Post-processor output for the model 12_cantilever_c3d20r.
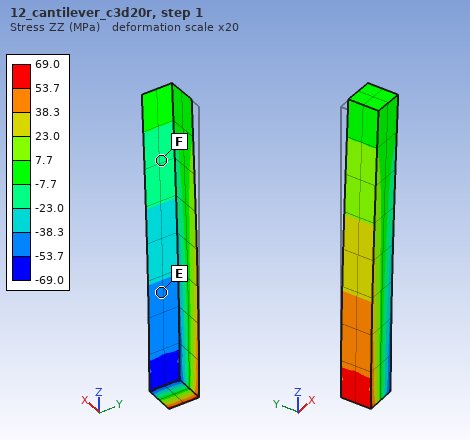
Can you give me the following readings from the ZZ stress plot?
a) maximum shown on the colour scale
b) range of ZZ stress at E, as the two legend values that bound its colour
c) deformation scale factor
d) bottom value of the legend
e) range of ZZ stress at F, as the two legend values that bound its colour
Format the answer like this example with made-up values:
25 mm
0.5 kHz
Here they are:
69.0 MPa
-53.7 to -38.3 MPa
20
-69.0 MPa
-23.0 to -7.7 MPa
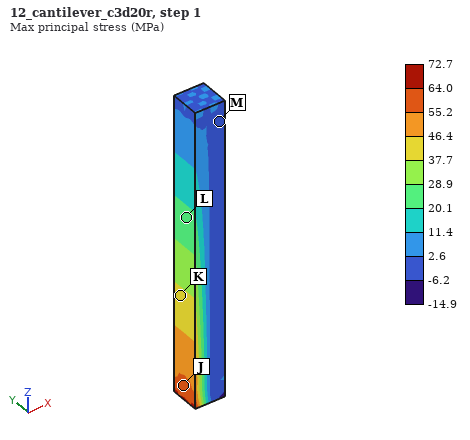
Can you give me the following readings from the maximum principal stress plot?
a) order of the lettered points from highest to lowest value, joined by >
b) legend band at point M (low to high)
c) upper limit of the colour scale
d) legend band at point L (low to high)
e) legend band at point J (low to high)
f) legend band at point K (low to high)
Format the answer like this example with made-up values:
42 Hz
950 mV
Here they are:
J > K > L > M
-6.2 to 2.6 MPa
72.7 MPa
20.1 to 28.9 MPa
55.2 to 64.0 MPa
37.7 to 46.4 MPa
